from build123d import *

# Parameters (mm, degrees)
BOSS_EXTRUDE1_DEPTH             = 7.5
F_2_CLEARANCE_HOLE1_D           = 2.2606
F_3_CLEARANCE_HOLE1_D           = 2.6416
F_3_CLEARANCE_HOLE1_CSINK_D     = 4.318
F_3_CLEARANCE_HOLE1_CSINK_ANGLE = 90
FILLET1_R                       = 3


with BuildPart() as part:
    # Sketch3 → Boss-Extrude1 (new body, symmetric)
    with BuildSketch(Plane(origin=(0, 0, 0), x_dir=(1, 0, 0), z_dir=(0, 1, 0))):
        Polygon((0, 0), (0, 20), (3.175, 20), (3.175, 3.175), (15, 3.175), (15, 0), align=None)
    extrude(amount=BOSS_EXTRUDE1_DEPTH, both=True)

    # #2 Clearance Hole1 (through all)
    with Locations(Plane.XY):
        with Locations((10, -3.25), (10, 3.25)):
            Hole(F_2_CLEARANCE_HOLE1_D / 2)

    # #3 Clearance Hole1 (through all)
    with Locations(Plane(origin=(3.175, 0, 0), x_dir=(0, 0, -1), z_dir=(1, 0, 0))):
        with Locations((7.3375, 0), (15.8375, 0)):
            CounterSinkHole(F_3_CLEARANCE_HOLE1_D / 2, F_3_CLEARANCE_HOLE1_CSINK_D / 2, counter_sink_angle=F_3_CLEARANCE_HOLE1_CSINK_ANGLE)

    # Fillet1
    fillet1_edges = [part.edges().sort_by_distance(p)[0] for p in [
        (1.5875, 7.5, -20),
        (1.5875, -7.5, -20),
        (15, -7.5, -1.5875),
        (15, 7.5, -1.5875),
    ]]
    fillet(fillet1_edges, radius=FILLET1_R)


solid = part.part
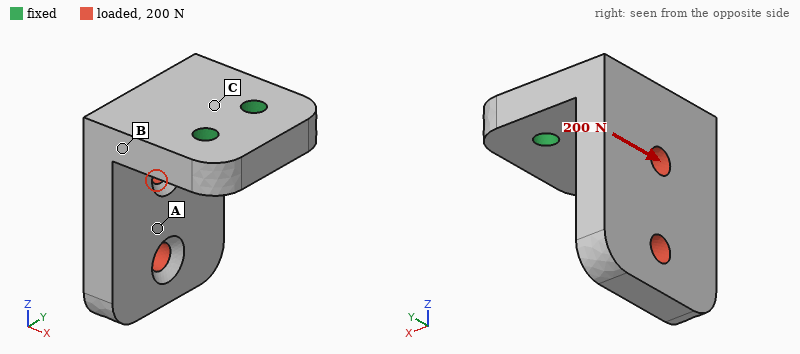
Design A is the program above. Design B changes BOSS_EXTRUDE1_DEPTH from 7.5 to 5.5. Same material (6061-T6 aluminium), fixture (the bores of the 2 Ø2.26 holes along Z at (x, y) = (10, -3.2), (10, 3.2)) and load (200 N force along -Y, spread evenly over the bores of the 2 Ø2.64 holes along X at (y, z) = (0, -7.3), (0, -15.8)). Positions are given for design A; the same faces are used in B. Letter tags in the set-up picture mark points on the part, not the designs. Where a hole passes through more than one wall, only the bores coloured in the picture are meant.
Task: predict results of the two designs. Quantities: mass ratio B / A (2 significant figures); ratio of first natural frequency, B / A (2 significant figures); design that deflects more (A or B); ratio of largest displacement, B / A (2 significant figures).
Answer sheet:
0.72
1.0
B
1.6
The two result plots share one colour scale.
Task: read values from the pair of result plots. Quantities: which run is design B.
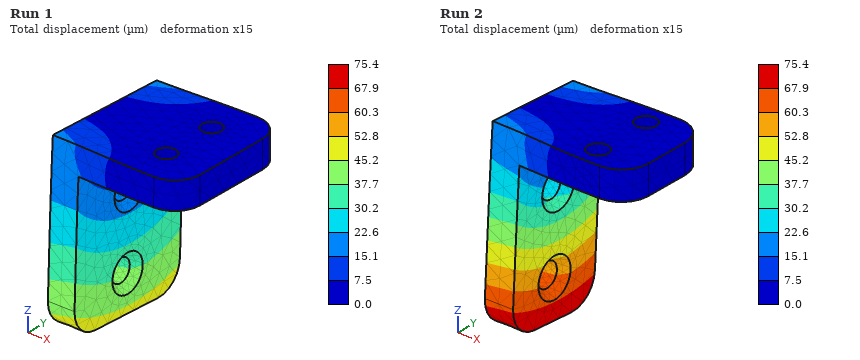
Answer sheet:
Run 2
